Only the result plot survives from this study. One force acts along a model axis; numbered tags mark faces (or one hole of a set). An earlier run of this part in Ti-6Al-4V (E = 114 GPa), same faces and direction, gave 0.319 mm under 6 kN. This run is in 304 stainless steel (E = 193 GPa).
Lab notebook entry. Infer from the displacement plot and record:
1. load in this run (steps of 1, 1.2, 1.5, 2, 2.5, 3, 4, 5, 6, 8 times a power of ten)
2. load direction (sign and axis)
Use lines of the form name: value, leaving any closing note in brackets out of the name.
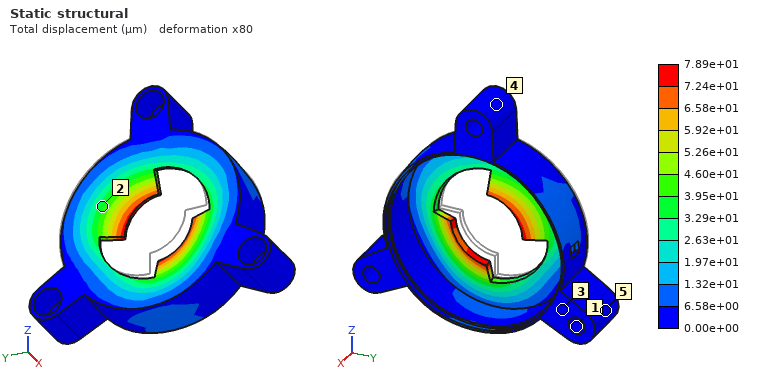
load in this run: 2.5 kN
load direction: +X
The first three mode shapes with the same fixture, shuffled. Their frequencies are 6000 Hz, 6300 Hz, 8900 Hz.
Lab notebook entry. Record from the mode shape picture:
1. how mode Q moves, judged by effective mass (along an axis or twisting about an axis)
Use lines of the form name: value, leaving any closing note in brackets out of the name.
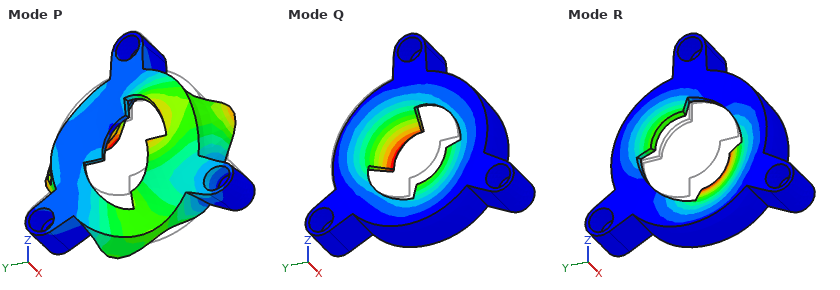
how mode Q moves, judged by effective mass: along X
